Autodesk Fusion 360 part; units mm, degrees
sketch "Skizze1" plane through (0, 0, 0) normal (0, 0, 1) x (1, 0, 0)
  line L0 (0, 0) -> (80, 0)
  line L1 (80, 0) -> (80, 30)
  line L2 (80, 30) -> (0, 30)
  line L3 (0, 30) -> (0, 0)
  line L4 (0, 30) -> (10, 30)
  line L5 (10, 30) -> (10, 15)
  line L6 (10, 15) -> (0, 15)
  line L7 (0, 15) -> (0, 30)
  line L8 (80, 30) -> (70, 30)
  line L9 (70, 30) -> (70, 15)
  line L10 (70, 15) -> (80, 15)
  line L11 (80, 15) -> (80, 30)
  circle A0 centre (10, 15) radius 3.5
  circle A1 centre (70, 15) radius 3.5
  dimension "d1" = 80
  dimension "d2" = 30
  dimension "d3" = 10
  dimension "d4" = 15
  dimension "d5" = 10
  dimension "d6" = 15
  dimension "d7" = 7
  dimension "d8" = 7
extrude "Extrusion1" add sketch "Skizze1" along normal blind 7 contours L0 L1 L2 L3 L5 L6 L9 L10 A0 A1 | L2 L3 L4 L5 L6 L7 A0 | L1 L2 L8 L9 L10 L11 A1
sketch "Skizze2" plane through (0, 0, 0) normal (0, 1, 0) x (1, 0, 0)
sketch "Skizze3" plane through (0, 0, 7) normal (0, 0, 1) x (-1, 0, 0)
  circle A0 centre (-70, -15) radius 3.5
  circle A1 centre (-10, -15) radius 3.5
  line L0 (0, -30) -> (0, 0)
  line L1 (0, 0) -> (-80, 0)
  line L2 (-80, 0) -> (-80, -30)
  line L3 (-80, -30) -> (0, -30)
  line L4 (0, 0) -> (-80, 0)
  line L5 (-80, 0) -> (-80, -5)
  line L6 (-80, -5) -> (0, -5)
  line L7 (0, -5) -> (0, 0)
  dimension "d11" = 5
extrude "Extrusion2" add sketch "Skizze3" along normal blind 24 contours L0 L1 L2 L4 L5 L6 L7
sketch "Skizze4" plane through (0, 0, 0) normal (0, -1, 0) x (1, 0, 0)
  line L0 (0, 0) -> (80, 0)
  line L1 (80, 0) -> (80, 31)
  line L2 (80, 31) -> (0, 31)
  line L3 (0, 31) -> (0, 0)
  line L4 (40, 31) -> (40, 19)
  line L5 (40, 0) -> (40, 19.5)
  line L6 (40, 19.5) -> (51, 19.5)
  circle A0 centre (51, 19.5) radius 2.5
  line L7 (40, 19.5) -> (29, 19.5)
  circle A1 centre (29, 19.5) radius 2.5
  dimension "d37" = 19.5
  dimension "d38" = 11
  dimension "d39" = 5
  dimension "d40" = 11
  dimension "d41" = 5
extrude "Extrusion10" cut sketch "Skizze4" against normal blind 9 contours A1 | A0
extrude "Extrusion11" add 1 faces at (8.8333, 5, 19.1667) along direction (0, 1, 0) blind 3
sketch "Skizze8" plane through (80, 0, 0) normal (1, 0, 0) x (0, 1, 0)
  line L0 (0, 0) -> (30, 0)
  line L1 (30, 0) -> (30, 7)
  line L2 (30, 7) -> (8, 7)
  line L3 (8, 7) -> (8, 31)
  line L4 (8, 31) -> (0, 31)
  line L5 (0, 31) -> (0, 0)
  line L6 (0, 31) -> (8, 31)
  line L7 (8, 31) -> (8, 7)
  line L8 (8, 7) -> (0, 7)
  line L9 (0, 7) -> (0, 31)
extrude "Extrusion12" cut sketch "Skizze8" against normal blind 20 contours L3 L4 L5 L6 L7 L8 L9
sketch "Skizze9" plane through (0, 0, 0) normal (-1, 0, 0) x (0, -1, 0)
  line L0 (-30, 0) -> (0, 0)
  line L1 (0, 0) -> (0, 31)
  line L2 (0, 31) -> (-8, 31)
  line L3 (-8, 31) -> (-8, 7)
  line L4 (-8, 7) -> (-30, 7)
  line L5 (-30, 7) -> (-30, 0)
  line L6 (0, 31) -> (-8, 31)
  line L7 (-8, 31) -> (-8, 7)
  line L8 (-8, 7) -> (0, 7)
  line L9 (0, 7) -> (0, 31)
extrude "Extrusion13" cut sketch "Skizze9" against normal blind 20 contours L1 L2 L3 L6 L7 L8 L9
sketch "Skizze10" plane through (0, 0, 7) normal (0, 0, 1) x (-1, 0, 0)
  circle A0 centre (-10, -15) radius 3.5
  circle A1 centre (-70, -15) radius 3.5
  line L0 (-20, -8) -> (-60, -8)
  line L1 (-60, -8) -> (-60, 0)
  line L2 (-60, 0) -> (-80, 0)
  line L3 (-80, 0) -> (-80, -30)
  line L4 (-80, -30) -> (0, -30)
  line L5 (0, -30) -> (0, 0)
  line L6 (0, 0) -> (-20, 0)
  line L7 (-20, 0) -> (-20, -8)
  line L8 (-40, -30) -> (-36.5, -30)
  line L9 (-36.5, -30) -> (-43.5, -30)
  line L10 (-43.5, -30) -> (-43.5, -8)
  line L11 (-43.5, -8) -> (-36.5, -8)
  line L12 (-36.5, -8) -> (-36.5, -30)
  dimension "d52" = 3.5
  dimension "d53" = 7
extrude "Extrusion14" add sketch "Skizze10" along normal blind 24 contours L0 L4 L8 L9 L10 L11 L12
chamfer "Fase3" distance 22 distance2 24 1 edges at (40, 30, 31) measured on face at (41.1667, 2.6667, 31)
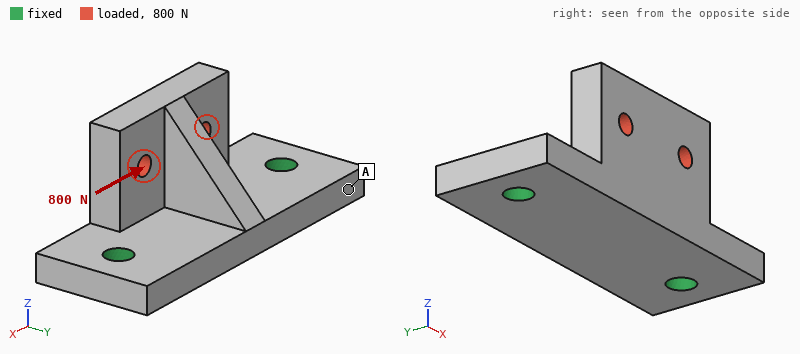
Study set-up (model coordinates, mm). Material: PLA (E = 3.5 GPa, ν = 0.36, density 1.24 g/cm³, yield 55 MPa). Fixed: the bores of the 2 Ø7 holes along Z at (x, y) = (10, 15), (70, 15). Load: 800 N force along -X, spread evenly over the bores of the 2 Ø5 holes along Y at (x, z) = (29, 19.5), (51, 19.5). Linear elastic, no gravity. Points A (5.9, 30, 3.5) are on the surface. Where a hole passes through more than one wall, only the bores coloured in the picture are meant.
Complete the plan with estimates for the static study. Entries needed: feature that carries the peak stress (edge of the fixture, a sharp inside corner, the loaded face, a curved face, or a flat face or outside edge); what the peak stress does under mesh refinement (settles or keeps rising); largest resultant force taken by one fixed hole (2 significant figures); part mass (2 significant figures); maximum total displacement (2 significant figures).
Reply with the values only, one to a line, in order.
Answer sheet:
edge of the fixture
keeps rising
500 N
32 g
0.17 mm
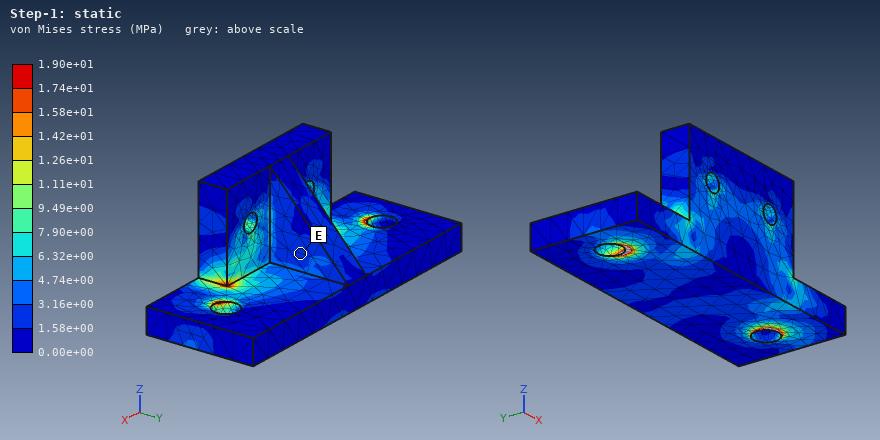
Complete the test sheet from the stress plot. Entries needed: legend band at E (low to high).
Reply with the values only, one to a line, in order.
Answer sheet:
1.58e+00 to 3.16e+00 MPa
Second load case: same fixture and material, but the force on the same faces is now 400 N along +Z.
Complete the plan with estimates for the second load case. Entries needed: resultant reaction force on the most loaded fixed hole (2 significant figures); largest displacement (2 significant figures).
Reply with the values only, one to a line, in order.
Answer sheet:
210 N
0.21 mm
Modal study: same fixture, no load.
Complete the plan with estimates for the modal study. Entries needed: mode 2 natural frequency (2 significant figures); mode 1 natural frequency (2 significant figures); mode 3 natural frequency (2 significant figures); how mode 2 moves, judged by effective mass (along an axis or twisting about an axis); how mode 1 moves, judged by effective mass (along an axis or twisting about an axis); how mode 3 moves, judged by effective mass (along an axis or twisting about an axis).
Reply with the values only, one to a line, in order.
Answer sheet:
2800 Hz
1600 Hz
3600 Hz
along Z
along Y
along X
